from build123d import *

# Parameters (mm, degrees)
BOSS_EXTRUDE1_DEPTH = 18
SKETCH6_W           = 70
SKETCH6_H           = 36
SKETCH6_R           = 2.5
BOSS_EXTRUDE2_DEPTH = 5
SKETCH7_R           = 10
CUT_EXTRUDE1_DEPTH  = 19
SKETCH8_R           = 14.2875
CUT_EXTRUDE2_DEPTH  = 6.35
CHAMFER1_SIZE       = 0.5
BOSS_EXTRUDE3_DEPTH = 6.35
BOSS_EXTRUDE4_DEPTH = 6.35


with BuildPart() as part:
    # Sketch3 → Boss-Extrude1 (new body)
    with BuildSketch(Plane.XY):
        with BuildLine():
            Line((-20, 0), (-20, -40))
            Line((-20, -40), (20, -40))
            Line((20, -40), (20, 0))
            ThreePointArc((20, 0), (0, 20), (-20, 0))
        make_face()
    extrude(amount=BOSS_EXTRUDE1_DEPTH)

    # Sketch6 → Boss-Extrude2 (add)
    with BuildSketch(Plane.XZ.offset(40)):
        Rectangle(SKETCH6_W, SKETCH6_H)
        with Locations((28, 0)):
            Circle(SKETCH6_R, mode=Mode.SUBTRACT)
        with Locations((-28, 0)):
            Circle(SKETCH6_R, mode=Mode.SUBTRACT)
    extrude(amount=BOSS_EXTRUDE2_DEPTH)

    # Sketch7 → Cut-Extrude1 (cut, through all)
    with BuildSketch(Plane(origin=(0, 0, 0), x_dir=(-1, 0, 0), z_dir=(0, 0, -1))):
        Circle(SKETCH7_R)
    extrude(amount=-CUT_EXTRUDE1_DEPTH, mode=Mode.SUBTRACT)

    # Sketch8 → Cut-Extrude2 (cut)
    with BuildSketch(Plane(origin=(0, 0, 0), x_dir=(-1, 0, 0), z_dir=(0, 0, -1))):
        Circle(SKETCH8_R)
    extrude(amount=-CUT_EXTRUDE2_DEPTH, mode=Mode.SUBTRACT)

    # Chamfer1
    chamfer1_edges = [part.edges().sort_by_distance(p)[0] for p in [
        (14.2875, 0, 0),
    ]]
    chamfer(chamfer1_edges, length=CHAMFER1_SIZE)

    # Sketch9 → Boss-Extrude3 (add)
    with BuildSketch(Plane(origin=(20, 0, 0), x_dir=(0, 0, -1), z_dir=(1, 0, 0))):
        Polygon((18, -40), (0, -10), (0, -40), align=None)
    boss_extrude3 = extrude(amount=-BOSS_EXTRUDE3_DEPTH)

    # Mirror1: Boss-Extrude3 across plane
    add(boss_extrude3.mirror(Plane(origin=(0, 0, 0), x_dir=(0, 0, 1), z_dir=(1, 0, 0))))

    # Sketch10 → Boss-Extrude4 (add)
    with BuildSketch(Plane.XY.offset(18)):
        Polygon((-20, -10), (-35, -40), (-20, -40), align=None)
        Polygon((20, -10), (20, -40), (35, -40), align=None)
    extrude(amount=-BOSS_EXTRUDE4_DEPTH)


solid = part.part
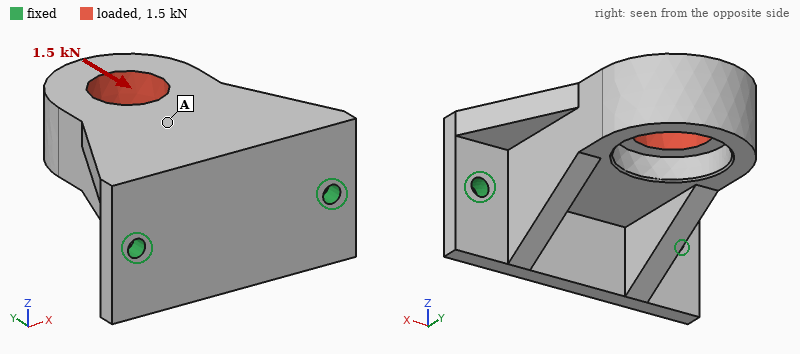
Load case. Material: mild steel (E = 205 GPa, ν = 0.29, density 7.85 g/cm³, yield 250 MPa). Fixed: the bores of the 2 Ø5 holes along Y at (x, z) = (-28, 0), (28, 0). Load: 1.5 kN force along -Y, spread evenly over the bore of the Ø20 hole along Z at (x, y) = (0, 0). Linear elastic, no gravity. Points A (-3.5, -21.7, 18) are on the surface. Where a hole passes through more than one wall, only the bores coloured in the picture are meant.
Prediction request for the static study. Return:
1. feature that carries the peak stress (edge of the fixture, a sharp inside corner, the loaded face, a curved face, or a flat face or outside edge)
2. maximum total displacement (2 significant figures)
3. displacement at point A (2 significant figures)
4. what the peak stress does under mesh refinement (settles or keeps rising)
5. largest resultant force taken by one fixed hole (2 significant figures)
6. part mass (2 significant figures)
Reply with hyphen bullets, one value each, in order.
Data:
- edge of the fixture
- 42 µm
- 19 µm
- keeps rising
- 790 N
- 400 g
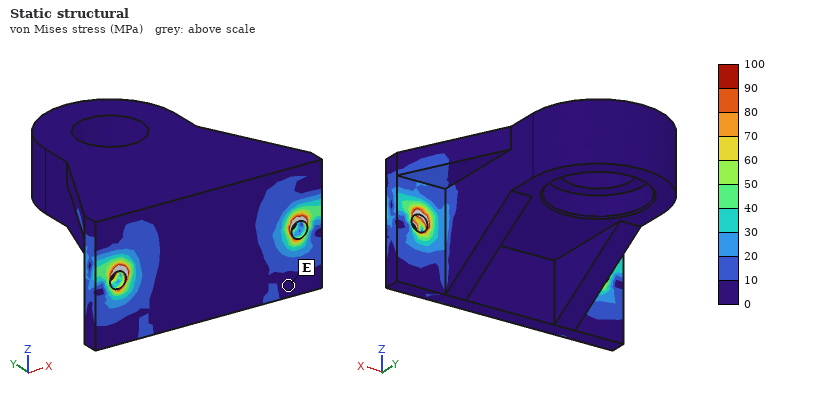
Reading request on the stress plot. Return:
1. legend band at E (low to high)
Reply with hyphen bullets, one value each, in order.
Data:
- 0 to 10 MPa
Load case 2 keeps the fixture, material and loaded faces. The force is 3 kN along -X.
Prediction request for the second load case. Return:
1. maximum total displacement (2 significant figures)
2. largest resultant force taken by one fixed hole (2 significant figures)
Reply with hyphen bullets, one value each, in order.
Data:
- 30 µm
- 3.0 kN
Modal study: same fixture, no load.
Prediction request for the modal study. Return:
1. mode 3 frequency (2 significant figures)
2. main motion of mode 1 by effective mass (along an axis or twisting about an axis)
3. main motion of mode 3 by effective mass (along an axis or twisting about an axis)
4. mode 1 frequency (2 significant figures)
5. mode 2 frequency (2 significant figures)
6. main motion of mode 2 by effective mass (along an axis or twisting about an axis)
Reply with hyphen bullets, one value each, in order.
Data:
- 6400 Hz
- along Z
- along Y
- 1400 Hz
- 4700 Hz
- along X
